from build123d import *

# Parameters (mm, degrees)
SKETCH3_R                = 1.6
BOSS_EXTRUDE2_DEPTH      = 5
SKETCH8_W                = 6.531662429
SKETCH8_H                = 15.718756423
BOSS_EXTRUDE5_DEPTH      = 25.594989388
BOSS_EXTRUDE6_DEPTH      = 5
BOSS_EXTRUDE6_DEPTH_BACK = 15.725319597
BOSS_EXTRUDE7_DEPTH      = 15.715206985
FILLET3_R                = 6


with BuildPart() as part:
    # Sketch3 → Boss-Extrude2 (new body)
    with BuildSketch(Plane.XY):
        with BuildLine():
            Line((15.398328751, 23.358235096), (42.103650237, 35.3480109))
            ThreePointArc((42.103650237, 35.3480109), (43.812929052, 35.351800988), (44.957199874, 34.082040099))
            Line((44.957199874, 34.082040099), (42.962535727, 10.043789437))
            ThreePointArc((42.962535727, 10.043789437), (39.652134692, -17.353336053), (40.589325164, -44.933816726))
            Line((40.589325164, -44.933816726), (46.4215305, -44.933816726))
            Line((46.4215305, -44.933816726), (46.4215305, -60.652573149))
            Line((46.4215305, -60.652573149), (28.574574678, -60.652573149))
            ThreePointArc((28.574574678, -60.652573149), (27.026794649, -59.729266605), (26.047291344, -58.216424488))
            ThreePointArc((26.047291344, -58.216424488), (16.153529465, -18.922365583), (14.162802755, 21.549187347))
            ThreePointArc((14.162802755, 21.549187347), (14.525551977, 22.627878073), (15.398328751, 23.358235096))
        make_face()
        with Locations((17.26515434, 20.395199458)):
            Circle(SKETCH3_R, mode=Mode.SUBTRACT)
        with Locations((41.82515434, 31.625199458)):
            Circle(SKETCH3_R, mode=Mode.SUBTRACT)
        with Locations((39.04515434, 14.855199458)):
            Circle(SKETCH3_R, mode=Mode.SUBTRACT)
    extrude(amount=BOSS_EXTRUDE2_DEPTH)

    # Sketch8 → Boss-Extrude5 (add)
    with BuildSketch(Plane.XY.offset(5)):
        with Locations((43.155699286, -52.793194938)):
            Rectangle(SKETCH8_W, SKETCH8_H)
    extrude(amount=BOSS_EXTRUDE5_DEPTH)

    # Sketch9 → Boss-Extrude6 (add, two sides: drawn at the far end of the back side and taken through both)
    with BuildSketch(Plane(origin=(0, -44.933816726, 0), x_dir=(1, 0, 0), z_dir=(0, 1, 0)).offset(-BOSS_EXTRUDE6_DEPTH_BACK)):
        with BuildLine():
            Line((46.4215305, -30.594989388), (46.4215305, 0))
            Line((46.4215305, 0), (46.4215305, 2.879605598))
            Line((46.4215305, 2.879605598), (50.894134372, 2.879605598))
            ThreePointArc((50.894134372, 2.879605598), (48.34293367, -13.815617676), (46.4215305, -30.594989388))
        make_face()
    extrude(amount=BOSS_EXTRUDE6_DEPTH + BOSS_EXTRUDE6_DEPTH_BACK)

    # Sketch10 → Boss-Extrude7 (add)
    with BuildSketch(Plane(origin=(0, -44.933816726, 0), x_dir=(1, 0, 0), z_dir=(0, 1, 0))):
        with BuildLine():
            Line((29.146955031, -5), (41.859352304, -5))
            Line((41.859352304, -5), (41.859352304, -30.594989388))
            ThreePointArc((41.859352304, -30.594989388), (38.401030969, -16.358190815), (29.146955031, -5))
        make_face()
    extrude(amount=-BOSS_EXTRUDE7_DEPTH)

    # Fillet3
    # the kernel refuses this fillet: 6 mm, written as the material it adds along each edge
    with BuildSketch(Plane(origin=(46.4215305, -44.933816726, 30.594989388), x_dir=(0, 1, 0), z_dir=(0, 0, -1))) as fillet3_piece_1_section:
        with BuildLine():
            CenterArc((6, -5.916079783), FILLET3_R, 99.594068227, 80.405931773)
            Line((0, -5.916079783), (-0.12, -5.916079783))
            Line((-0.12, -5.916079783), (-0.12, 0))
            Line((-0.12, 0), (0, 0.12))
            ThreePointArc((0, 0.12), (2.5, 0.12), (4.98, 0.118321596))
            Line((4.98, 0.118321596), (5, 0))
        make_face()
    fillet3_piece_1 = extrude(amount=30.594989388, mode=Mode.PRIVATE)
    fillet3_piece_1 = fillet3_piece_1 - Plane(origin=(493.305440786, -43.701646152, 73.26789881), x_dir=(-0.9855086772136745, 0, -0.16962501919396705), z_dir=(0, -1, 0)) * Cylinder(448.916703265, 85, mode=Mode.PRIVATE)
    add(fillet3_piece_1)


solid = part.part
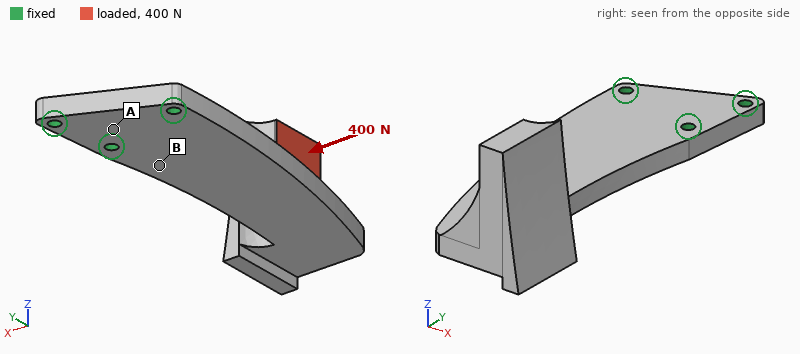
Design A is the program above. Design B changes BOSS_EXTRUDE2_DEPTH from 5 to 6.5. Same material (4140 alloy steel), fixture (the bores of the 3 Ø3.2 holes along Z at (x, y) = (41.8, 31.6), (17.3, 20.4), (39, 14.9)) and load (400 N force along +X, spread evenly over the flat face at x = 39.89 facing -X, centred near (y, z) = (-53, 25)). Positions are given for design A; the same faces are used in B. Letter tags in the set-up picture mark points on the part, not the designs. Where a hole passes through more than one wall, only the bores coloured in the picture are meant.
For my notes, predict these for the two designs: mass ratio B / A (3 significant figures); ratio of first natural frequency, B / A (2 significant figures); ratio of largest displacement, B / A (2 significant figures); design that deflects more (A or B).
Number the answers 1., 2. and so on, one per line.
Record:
1. 1.18
2. 1.4
3. 0.52
4. A
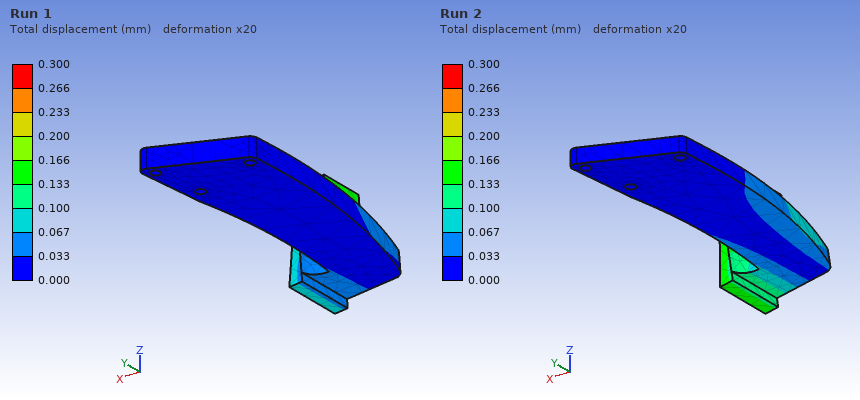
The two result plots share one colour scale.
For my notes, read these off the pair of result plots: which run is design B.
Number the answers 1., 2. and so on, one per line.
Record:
1. Run 1
